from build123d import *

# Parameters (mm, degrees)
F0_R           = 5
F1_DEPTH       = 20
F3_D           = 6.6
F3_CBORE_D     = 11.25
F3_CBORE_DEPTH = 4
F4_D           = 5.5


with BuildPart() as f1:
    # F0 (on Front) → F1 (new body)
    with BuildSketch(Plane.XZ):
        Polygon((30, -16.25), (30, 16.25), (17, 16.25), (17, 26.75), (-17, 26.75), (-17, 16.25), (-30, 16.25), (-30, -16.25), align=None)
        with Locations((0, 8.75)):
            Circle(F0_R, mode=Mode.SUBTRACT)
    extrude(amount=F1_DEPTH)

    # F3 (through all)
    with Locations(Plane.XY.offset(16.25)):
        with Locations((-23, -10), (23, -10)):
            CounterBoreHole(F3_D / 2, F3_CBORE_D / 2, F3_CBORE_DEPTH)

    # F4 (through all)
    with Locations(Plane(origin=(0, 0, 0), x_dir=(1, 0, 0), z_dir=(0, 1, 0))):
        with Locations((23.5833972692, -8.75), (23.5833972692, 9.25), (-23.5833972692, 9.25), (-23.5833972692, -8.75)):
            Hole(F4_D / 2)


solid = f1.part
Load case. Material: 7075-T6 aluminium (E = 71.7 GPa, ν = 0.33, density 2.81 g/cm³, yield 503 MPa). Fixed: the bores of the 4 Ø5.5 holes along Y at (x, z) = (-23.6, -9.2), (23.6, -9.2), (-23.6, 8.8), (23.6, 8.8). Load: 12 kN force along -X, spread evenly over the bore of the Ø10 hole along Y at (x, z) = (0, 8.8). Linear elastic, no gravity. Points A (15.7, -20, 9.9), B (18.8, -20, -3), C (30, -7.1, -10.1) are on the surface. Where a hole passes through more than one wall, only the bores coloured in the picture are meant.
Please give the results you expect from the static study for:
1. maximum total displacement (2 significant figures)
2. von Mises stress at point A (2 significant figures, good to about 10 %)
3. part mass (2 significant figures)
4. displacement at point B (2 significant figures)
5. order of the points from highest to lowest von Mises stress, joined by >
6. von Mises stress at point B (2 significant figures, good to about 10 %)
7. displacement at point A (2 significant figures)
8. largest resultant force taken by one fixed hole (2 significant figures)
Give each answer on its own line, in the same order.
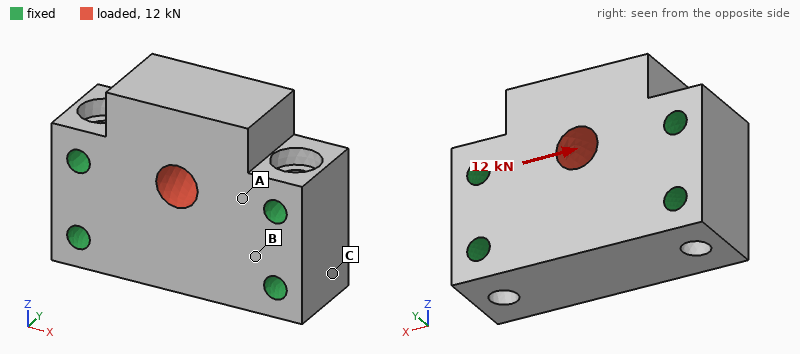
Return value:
6.2 µm
22 MPa
110 g
0.94 µm
A > B > C
8.5 MPa
2.0 µm
4.3 kN
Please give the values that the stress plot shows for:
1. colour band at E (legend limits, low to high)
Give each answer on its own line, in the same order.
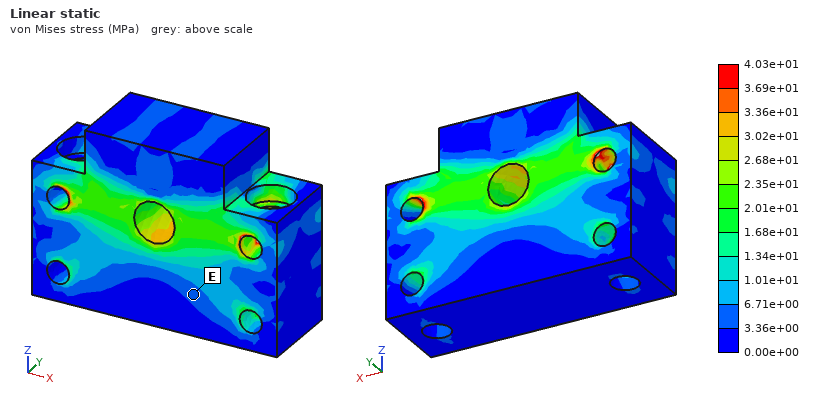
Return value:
3.36e+00 to 6.71e+00 MPa
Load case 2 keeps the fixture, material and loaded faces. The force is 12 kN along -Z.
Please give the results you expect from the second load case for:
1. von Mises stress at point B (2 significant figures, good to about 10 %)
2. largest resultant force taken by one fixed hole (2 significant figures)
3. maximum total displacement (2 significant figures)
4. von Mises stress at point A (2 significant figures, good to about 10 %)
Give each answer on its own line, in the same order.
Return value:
22 MPa
3.5 kN
10 µm
17 MPa
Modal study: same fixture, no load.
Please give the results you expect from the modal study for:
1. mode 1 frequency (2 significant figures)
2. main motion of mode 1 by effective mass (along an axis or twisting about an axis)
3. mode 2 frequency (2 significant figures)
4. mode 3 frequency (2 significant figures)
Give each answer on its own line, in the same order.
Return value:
17 kHz
along Y
26 kHz
26 kHz
